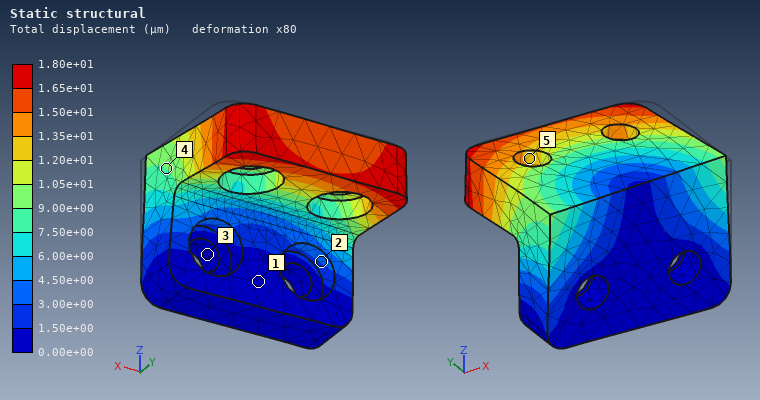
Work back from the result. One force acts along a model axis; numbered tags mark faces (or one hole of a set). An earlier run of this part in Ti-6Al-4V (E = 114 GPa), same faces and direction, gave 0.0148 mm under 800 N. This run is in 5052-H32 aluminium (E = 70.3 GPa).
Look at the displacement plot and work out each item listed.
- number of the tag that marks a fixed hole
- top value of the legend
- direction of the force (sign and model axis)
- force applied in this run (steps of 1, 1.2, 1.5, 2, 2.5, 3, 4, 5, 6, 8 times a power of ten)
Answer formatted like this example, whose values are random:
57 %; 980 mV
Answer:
3; 1.80e+01 µm; -X; 600 N
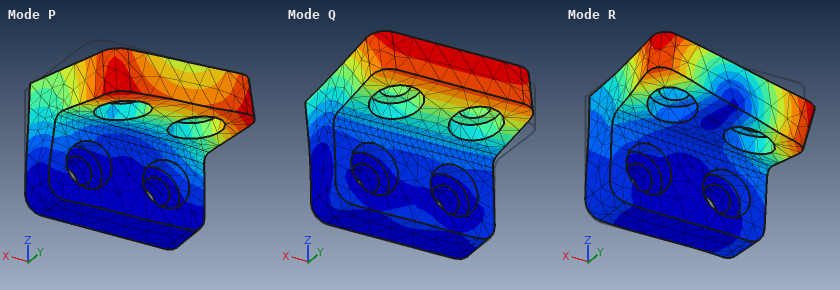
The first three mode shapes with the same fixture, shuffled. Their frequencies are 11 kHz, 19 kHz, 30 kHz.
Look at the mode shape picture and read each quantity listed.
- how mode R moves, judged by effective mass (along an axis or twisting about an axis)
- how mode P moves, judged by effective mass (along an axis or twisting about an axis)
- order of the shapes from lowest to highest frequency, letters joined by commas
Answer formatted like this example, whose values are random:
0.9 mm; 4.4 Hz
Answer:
along X; along X; Q, P, R
